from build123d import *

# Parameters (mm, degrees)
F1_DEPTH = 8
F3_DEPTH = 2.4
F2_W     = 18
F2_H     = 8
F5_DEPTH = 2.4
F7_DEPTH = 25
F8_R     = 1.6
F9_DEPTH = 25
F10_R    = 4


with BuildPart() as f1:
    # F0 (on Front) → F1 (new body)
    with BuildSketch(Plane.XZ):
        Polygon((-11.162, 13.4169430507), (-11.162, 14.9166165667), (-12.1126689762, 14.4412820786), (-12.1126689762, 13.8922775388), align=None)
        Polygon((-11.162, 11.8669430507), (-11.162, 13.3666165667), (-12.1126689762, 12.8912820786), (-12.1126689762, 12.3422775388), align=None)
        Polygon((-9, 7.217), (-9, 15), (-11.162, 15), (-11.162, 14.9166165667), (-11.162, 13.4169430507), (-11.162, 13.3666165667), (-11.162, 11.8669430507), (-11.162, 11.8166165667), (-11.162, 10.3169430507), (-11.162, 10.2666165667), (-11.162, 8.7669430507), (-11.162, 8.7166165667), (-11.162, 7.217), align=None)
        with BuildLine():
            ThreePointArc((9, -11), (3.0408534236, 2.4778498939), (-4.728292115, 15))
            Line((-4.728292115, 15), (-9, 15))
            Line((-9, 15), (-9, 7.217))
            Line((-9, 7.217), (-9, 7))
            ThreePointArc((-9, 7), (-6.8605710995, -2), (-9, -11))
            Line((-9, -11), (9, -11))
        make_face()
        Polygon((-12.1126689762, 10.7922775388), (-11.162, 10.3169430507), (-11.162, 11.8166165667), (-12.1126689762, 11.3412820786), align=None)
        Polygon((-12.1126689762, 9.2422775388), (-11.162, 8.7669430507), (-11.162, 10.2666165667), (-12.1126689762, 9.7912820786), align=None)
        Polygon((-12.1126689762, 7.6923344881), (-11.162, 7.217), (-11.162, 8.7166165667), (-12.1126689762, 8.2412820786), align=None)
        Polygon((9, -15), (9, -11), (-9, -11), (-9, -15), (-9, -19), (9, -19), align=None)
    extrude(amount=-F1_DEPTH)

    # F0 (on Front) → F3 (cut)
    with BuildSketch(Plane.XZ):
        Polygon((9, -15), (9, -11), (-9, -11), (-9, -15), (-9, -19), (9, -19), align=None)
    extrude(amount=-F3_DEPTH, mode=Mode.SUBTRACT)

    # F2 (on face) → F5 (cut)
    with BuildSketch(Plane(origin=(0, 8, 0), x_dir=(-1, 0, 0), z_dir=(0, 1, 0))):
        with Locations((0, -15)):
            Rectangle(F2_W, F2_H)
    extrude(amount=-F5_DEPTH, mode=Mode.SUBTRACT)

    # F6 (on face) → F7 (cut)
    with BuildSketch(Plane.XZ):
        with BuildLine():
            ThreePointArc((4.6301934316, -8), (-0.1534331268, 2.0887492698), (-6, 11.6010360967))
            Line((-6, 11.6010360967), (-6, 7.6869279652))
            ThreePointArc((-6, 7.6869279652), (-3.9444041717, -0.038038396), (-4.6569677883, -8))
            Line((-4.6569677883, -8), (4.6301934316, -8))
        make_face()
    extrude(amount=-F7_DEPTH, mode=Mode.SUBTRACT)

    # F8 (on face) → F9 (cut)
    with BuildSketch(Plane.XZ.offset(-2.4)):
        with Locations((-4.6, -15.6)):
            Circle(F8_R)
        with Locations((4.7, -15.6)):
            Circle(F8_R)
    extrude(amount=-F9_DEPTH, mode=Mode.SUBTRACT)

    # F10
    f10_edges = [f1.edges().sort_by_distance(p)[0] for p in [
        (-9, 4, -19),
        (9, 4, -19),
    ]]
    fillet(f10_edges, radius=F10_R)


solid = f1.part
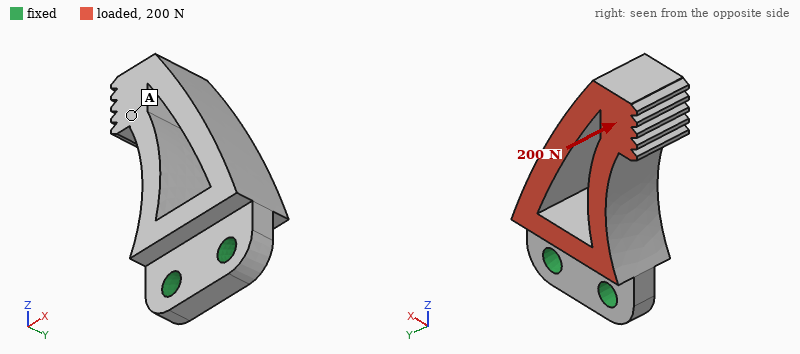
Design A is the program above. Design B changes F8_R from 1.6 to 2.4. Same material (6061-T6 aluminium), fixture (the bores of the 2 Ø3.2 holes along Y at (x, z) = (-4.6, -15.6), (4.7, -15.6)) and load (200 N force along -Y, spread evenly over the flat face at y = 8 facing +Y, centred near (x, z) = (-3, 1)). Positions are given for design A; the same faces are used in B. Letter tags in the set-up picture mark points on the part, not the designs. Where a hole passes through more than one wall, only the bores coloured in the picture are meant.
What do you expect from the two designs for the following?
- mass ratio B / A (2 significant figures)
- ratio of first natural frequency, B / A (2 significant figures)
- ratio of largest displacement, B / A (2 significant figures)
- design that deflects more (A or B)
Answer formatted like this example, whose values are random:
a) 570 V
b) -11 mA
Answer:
a) 0.97
b) 1.1
c) 0.80
d) A
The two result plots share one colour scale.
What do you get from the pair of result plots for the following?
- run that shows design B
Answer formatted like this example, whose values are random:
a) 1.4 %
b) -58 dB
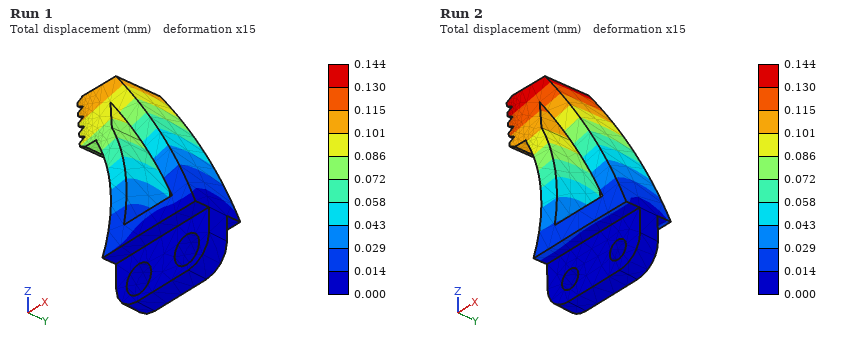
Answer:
a) Run 1
